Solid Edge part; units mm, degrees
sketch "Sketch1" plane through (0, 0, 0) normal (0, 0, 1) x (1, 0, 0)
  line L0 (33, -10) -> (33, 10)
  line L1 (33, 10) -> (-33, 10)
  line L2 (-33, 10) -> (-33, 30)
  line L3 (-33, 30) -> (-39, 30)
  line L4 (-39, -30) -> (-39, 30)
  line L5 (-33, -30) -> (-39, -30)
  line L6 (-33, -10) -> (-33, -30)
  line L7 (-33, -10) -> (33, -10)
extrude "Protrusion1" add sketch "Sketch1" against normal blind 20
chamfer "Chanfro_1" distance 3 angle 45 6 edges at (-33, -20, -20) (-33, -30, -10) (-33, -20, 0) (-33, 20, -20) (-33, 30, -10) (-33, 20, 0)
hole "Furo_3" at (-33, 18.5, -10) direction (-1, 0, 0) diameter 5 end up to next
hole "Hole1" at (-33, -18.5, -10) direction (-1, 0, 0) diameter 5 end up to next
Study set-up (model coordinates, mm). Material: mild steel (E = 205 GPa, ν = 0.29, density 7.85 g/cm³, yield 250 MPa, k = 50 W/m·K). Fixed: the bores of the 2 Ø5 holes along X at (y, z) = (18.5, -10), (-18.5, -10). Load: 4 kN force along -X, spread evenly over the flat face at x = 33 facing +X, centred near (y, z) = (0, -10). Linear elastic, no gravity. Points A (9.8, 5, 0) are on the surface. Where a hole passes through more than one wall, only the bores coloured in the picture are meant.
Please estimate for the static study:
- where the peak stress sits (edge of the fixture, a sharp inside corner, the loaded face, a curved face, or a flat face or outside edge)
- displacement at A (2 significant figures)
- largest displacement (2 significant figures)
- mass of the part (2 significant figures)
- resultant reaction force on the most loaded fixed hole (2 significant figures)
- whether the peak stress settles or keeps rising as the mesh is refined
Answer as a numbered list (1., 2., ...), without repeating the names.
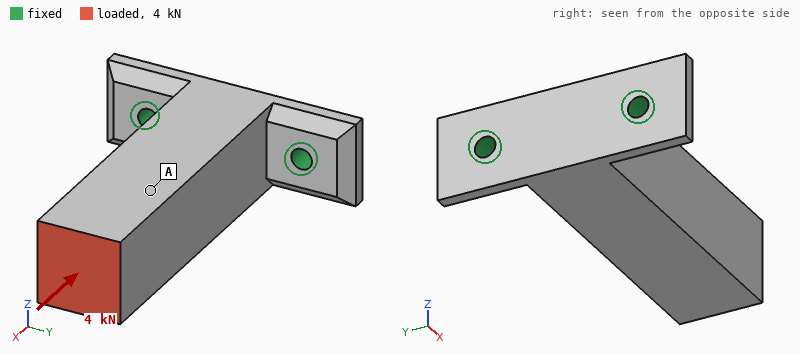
1. edge of the fixture
2. 8.3 µm
3. 9.5 µm
4. 260 g
5. 2.1 kN
6. keeps rising
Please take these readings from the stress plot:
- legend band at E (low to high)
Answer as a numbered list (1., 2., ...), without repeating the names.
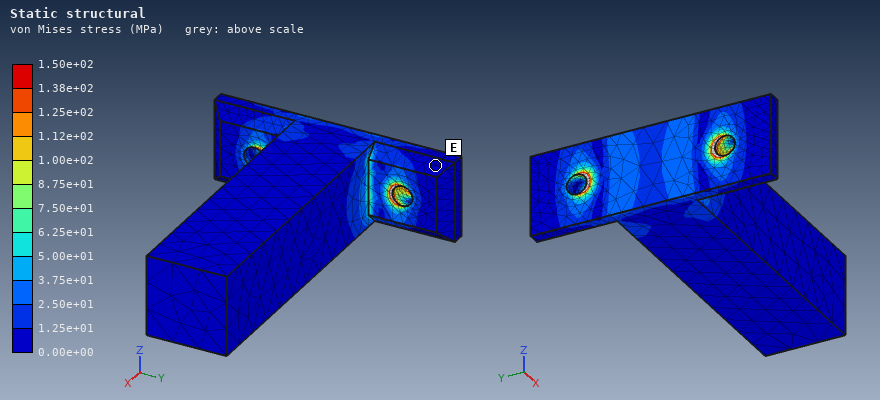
1. 0.00e+00 to 1.25e+01 MPa
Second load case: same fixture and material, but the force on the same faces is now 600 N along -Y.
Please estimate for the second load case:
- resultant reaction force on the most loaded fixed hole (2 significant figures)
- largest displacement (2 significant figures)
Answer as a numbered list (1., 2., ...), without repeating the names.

1. 1.5 kN
2. 46 µm
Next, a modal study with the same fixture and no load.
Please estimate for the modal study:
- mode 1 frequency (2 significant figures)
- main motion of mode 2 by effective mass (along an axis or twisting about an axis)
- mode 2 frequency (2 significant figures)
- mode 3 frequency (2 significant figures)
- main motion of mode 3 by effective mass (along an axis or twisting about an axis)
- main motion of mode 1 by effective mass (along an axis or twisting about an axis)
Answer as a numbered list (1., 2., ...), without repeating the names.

1. 1200 Hz
2. along Y
3. 2300 Hz
4. 7800 Hz
5. along X
6. along Z
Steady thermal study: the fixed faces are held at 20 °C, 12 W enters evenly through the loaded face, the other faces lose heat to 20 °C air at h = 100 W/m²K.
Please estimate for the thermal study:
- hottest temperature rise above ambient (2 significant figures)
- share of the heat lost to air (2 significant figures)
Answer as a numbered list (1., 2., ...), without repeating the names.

1. 28 K
2. 67 %
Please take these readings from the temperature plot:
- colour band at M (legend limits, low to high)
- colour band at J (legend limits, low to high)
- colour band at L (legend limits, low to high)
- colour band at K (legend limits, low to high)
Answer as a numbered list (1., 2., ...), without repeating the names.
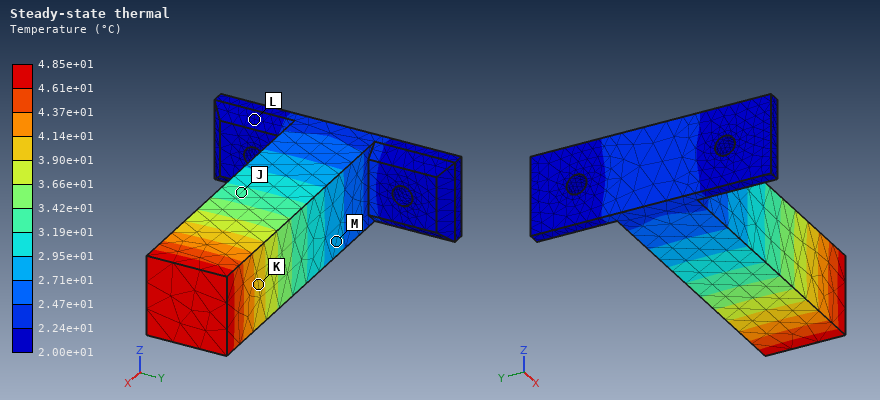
1. 2.71e+01 to 2.95e+01 °C
2. 3.19e+01 to 3.42e+01 °C
3. 2.00e+01 to 2.24e+01 °C
4. 3.90e+01 to 4.14e+01 °C
